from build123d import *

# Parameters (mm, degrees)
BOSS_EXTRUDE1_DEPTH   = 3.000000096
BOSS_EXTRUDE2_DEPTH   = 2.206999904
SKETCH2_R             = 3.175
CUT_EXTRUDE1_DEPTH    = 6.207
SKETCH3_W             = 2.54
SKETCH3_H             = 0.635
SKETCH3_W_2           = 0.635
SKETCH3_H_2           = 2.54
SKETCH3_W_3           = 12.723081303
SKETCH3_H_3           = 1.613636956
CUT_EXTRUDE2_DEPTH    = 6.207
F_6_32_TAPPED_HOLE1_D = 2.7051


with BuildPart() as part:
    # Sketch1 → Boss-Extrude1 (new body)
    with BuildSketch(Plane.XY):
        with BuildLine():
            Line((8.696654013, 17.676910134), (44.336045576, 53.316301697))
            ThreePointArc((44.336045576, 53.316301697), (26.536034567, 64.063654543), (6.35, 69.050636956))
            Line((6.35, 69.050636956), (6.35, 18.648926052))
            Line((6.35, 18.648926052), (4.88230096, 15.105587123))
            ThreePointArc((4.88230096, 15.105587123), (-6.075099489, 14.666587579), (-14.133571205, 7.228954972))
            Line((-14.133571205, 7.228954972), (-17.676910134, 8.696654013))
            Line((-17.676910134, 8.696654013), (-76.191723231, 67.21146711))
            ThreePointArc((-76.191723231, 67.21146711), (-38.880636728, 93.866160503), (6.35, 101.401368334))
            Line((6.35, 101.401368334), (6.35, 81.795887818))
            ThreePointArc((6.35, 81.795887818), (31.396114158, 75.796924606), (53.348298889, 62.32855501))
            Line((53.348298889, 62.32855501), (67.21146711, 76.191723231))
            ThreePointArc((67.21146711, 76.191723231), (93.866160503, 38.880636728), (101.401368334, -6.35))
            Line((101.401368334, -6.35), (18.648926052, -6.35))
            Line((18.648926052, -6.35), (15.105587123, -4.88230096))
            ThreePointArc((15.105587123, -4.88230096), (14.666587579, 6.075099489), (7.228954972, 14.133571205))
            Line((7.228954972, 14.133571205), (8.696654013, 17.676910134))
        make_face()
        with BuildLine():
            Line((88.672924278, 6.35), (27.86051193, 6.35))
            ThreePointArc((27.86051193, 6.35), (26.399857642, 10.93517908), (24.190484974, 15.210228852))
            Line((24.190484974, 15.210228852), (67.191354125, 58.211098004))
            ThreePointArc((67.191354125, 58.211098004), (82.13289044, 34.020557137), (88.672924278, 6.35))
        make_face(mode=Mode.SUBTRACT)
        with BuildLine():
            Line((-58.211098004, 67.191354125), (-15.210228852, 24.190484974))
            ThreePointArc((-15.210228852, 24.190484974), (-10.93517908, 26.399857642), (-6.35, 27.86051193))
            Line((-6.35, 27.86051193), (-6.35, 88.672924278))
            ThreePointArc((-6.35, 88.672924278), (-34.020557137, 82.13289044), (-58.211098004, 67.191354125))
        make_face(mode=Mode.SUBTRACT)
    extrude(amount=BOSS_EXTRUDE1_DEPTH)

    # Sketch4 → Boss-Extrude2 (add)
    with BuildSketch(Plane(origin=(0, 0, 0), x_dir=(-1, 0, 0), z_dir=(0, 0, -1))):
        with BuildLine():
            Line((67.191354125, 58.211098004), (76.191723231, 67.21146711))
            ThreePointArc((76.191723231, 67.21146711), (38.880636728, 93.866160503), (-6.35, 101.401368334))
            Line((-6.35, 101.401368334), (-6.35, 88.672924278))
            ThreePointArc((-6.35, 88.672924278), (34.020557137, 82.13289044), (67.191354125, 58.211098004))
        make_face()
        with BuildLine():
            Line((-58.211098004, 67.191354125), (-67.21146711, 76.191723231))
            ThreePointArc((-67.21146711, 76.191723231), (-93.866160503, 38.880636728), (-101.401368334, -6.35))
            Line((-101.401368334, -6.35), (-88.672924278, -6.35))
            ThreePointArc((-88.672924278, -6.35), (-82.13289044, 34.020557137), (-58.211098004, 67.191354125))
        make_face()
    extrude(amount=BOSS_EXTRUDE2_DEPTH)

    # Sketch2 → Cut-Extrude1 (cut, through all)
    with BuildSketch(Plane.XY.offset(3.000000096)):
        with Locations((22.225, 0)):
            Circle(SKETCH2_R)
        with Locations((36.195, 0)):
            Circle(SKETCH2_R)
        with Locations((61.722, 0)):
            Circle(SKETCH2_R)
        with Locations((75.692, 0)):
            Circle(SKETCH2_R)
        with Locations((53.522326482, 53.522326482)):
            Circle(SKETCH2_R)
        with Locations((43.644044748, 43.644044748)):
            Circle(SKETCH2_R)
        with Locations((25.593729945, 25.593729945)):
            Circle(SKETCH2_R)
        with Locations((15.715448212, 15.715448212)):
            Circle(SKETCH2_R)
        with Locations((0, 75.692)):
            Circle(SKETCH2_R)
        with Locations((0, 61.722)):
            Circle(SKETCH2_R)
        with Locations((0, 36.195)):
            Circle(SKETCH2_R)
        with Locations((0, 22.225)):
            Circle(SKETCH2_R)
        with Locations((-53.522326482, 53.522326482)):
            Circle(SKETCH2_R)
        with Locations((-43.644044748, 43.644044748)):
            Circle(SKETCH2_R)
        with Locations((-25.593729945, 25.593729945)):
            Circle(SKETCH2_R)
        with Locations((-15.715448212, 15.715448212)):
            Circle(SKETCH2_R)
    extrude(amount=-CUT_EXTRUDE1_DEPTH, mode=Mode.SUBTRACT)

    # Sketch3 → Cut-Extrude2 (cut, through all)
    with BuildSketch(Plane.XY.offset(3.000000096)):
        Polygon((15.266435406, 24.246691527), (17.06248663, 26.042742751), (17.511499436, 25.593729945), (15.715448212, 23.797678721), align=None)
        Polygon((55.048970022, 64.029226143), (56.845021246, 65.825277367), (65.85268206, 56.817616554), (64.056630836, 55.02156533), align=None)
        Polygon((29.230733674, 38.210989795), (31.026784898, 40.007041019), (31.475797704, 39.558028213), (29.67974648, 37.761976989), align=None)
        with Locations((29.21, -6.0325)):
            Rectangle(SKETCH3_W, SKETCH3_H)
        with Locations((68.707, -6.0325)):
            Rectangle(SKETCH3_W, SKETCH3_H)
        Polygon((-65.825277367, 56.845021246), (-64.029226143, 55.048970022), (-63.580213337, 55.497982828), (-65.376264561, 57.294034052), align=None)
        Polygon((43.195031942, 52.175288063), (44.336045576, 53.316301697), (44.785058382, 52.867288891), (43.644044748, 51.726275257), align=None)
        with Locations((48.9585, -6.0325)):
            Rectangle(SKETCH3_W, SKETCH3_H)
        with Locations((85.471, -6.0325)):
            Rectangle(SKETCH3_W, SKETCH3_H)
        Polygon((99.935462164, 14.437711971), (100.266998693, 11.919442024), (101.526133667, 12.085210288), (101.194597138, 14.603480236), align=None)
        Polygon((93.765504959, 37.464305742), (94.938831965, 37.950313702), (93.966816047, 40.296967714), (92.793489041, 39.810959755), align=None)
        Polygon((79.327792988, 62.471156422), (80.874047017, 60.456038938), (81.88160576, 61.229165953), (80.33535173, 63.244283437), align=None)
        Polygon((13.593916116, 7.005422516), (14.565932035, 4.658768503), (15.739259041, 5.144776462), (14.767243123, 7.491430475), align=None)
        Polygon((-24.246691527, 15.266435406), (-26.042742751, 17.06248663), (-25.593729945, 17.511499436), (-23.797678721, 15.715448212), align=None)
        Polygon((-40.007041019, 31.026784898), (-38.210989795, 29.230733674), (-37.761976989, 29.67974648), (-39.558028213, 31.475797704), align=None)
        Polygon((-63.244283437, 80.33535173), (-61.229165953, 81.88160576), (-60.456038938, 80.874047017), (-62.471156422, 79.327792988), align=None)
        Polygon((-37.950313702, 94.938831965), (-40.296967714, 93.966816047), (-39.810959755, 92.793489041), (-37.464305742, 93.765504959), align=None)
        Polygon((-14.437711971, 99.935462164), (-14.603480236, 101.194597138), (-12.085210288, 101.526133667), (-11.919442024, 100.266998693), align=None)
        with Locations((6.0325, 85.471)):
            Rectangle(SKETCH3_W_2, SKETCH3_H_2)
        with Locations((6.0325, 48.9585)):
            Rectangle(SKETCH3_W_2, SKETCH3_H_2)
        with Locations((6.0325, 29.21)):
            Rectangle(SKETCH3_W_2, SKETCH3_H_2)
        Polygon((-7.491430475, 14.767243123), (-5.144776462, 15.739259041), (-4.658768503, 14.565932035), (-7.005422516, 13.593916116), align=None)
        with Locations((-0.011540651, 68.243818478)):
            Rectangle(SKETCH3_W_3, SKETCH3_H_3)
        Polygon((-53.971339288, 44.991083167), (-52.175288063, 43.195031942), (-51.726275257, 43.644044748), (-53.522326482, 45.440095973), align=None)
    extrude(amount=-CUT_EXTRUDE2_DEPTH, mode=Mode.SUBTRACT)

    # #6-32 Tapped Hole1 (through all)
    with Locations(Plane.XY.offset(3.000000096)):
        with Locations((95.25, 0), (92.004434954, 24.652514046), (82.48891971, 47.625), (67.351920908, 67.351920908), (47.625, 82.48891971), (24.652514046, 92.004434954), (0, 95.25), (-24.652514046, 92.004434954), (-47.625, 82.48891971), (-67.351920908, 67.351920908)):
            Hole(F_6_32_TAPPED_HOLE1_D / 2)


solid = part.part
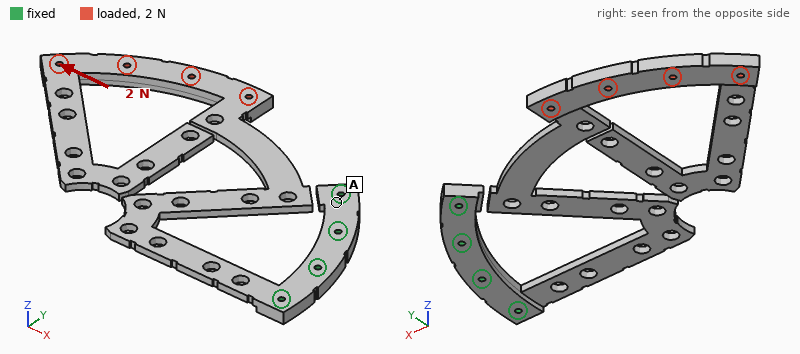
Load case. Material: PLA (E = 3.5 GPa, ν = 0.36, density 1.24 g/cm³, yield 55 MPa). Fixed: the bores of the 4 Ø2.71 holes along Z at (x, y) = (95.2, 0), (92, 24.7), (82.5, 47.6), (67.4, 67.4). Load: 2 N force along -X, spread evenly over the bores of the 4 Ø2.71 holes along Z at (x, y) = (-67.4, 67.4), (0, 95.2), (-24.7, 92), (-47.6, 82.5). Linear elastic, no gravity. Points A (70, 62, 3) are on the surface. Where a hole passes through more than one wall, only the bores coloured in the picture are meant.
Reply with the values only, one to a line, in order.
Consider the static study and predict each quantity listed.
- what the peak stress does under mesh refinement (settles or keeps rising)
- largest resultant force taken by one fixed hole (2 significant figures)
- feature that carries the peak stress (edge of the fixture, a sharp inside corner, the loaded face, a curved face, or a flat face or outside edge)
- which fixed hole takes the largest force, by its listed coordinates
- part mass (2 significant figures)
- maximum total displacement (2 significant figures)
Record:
keeps rising
6.9 N
a sharp inside corner
(92, 24.7)
28 g
2.0 mm
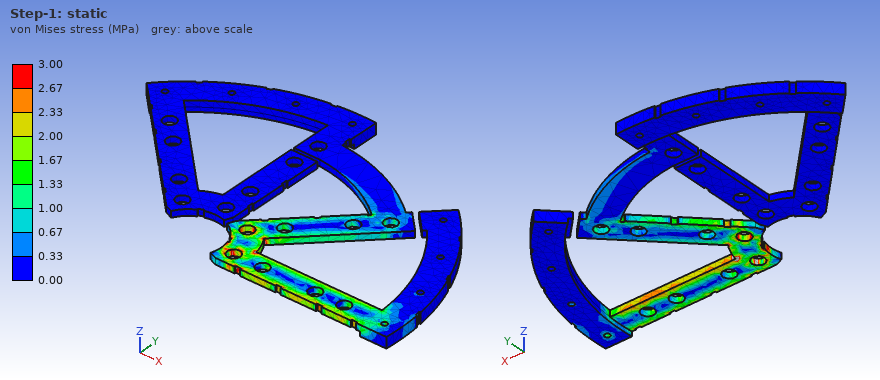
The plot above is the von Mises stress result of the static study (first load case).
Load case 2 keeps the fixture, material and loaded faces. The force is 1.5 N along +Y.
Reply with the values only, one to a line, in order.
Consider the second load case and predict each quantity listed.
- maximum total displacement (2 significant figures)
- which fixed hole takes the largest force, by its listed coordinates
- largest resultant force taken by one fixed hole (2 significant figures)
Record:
2.0 mm
(92, 24.7)
7.9 N
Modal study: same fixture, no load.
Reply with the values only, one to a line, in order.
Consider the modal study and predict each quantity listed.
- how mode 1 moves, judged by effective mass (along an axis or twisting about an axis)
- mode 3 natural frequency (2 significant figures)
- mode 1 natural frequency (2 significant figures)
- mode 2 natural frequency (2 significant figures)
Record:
along Z
42 Hz
11 Hz
33 Hz
